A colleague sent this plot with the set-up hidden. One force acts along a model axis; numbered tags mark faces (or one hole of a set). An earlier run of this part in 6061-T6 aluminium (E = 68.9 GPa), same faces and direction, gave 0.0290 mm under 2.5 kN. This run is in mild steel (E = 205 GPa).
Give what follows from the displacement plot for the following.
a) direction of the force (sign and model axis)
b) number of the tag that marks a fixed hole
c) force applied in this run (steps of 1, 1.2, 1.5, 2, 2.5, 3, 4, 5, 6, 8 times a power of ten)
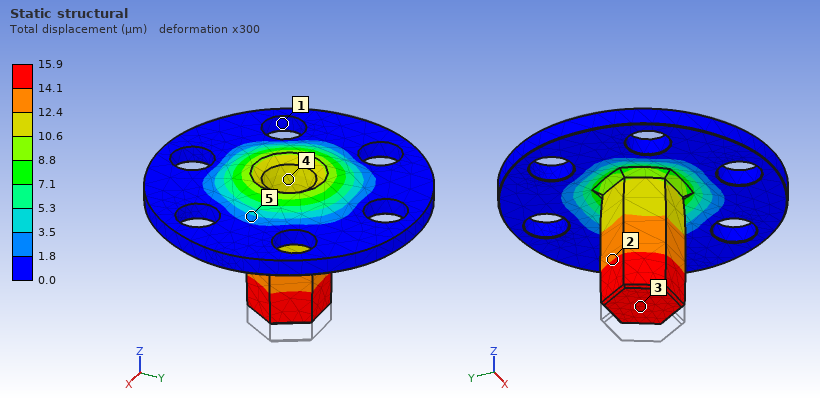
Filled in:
+Z
1
4 kN
